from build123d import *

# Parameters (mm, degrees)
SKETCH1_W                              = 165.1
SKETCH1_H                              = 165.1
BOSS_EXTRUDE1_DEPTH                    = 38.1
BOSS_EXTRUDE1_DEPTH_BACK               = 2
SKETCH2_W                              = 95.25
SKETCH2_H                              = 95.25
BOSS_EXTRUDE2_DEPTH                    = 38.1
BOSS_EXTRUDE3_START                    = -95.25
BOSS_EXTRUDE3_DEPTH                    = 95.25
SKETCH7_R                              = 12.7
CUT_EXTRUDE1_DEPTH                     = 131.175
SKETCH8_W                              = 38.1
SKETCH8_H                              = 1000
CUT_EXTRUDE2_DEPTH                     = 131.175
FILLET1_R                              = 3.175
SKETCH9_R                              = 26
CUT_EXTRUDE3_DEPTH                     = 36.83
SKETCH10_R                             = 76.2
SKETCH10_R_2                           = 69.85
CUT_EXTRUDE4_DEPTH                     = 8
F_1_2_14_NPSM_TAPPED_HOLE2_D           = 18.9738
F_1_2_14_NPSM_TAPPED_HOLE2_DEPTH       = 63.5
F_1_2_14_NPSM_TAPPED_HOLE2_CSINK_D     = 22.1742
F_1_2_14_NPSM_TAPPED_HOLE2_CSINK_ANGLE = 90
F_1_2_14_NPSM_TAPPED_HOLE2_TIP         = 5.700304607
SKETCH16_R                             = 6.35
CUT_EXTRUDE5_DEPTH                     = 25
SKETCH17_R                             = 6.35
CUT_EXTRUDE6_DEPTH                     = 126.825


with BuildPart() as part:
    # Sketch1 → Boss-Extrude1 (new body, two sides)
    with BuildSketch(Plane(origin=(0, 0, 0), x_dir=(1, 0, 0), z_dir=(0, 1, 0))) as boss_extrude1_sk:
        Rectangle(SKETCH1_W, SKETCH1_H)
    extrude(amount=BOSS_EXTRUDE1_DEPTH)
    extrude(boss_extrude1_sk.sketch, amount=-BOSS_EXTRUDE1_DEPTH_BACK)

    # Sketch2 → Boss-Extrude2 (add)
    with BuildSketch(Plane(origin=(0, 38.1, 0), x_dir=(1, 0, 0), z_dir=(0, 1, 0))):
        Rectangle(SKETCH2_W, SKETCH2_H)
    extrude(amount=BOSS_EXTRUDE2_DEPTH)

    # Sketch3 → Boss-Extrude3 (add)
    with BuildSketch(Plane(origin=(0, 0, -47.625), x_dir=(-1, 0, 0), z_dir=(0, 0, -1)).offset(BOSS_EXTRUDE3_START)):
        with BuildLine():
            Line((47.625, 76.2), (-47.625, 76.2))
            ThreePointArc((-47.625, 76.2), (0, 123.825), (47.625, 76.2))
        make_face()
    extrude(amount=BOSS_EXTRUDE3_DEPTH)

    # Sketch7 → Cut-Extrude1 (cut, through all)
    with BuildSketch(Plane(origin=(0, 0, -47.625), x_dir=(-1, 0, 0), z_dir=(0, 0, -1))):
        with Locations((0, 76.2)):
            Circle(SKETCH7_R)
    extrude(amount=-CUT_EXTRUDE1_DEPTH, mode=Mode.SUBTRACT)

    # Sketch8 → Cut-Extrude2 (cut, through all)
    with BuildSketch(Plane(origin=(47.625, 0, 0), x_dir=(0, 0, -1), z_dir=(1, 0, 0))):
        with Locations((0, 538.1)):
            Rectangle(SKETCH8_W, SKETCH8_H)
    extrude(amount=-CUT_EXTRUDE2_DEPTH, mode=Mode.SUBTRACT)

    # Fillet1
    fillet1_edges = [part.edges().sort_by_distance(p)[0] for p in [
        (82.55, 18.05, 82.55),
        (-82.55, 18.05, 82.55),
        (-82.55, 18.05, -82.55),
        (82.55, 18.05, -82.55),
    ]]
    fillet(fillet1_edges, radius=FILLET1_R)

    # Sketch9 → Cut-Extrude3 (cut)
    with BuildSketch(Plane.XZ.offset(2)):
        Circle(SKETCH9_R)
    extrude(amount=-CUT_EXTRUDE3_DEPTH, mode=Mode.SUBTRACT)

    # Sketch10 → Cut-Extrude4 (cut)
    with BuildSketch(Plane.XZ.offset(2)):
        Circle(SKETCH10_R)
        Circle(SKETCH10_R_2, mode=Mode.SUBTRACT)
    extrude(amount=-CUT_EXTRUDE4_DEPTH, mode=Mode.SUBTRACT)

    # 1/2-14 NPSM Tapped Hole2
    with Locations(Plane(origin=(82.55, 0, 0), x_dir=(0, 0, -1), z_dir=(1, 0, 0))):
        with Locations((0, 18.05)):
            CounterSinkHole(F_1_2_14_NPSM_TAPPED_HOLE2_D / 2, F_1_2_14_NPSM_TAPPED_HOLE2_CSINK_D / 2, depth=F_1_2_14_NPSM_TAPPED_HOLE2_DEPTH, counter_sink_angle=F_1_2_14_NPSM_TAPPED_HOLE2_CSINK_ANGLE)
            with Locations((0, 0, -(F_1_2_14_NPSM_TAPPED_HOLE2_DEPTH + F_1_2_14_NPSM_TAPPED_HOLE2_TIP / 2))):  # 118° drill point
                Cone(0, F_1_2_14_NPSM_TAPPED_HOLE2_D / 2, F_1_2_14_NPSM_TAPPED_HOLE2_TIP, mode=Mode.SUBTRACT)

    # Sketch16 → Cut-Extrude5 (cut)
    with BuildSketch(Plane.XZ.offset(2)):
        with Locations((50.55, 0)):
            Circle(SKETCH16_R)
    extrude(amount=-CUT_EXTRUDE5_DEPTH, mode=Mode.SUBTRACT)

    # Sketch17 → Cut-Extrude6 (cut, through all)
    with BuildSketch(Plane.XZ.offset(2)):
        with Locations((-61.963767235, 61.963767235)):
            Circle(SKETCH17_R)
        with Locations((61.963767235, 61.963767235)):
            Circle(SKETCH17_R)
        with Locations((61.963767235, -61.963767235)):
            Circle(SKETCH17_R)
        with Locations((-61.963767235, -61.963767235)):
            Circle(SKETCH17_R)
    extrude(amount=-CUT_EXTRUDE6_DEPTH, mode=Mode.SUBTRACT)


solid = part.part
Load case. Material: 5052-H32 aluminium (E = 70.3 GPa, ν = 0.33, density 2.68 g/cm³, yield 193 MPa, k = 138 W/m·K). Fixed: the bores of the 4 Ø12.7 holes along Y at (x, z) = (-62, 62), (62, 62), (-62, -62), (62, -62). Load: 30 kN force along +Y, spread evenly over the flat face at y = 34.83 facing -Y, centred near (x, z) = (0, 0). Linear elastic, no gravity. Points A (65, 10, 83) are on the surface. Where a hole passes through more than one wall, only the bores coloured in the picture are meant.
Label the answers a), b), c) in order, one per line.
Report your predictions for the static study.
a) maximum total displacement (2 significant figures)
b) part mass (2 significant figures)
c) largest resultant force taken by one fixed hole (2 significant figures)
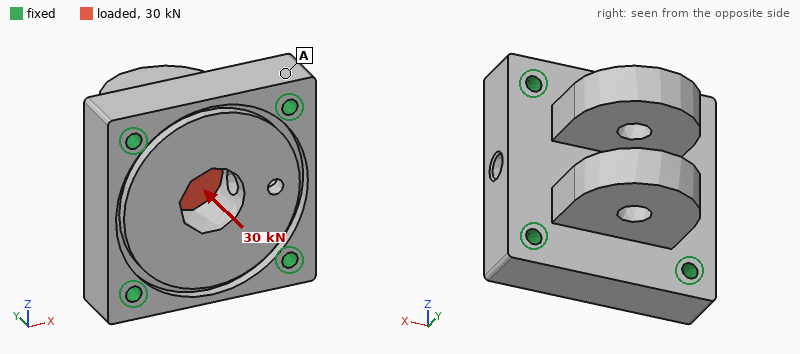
a) 0.20 mm
b) 3.6 kg
c) 7.7 kN
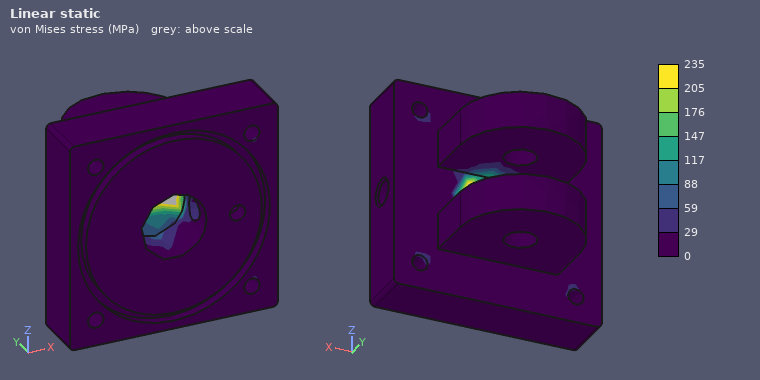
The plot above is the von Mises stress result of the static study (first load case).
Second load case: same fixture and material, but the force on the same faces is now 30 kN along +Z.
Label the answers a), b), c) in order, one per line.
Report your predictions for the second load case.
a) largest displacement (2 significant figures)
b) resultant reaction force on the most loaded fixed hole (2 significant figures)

a) 24 µm
b) 8.7 kN
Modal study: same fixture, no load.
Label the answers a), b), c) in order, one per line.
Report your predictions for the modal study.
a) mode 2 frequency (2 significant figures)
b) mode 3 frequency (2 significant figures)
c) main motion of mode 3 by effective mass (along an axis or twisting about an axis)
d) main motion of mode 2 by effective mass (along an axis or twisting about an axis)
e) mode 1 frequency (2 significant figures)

a) 2700 Hz
b) 4800 Hz
c) along X
d) along Z
e) 2600 Hz
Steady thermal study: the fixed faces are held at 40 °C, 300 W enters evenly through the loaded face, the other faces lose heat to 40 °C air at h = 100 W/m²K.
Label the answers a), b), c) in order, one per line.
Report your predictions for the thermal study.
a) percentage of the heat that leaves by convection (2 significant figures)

a) 28 %
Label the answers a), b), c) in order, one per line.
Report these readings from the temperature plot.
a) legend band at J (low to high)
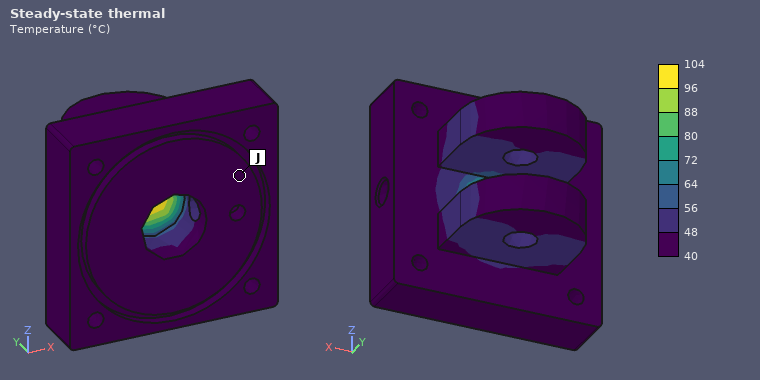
a) 40 to 48 °C
